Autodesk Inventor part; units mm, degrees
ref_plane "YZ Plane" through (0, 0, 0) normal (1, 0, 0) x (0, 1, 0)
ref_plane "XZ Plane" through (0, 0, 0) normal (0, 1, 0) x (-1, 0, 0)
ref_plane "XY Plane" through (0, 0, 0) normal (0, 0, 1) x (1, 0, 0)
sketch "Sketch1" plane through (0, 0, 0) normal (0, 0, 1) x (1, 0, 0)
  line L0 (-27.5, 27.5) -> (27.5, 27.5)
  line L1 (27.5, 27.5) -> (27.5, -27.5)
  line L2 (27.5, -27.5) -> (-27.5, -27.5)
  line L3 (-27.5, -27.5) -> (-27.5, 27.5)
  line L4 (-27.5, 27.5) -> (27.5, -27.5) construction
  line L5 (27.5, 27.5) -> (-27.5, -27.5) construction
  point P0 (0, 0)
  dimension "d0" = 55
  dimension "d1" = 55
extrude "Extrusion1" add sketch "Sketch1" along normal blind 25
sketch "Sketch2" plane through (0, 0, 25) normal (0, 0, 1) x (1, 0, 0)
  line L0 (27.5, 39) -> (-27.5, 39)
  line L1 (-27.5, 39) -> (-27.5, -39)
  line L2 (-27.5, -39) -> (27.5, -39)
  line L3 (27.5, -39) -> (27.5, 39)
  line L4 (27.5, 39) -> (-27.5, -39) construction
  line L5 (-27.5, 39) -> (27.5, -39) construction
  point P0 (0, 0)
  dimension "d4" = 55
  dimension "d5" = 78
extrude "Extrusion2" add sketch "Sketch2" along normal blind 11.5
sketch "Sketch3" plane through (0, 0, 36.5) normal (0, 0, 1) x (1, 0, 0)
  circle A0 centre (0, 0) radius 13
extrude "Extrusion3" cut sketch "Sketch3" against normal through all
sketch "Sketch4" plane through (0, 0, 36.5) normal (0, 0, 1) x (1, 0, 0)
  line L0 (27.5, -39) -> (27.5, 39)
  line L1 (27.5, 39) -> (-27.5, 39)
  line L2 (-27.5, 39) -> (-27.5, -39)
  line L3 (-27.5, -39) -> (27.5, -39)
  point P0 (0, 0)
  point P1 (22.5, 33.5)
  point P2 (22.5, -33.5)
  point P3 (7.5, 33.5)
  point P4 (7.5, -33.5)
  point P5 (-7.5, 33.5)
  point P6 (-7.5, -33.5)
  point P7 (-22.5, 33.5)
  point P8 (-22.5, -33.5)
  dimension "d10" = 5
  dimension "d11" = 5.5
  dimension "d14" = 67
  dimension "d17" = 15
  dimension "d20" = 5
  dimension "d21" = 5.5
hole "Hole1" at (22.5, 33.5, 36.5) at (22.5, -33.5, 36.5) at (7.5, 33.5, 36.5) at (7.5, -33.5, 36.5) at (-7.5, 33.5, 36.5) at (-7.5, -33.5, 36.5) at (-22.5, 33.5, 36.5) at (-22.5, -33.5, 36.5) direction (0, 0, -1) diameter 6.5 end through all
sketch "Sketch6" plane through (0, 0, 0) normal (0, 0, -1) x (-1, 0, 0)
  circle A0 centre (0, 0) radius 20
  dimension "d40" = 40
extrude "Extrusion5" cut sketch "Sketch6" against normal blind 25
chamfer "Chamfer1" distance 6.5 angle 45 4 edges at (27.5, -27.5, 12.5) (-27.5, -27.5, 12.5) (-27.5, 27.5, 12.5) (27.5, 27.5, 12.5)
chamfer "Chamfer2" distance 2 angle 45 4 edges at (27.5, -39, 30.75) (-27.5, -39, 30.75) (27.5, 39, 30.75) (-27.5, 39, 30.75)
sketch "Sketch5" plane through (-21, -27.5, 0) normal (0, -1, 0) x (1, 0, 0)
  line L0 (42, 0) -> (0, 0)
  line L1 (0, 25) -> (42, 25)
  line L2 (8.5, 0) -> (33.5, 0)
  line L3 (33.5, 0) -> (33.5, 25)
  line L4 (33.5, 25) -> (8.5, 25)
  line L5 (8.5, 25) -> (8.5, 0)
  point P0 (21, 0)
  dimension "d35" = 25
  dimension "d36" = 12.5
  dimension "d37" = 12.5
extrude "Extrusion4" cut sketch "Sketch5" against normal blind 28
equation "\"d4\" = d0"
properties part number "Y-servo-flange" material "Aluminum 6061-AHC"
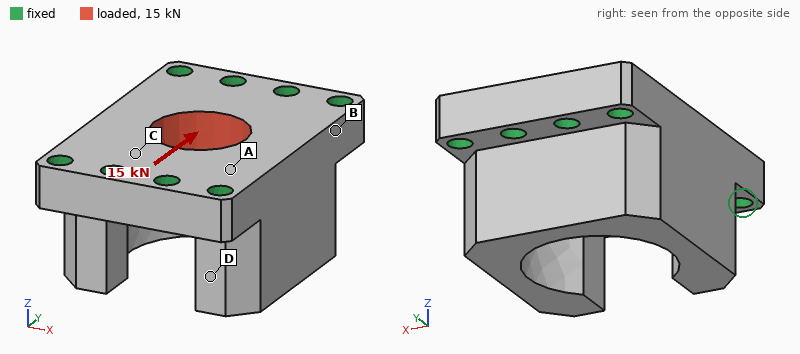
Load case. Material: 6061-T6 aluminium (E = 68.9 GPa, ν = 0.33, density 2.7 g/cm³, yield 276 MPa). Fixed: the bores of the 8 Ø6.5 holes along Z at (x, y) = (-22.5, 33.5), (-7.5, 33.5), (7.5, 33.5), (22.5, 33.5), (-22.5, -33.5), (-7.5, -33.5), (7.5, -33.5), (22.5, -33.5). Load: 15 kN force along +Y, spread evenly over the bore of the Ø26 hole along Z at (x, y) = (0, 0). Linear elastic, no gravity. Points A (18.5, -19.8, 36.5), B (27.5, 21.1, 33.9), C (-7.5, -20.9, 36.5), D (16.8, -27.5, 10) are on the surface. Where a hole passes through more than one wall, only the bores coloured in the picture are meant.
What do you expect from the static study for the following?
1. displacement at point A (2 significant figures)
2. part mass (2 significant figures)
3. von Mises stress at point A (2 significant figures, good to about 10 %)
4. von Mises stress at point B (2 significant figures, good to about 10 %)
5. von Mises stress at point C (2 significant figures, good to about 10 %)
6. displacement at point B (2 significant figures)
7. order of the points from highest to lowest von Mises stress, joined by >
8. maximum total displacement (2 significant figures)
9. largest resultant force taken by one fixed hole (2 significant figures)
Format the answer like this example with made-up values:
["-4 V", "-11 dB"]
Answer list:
["2.0 µm", "210 g", "11 MPa", "5.5 MPa", "16 MPa", "2.0 µm", "C > A > B > D", "5.9 µm", "2.2 kN"]
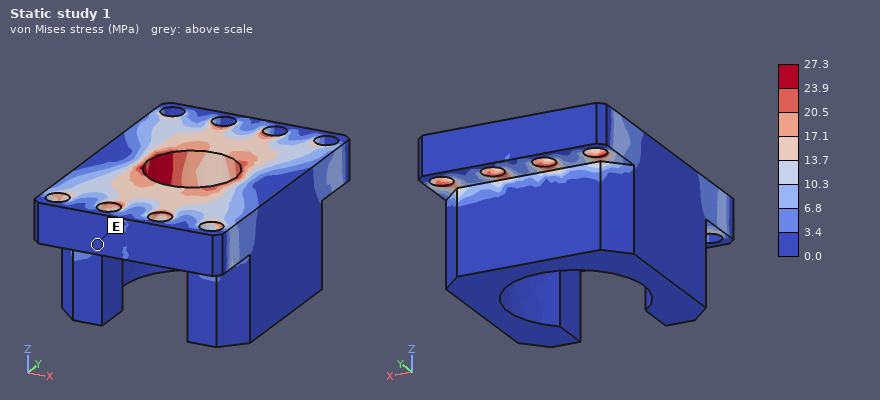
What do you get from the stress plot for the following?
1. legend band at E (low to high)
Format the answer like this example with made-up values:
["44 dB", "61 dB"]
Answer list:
["0.0 to 3.4 MPa"]
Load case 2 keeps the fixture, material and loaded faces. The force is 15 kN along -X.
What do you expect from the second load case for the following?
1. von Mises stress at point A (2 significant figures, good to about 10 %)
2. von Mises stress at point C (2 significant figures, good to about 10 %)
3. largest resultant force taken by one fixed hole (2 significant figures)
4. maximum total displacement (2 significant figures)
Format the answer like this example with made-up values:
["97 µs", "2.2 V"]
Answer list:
["22 MPa", "21 MPa", "2.6 kN", "17 µm"]
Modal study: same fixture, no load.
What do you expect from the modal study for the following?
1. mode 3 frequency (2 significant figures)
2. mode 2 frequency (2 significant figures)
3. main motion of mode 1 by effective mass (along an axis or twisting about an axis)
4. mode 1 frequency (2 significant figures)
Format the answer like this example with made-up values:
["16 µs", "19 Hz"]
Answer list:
["14 kHz", "9400 Hz", "along X", "9000 Hz"]
